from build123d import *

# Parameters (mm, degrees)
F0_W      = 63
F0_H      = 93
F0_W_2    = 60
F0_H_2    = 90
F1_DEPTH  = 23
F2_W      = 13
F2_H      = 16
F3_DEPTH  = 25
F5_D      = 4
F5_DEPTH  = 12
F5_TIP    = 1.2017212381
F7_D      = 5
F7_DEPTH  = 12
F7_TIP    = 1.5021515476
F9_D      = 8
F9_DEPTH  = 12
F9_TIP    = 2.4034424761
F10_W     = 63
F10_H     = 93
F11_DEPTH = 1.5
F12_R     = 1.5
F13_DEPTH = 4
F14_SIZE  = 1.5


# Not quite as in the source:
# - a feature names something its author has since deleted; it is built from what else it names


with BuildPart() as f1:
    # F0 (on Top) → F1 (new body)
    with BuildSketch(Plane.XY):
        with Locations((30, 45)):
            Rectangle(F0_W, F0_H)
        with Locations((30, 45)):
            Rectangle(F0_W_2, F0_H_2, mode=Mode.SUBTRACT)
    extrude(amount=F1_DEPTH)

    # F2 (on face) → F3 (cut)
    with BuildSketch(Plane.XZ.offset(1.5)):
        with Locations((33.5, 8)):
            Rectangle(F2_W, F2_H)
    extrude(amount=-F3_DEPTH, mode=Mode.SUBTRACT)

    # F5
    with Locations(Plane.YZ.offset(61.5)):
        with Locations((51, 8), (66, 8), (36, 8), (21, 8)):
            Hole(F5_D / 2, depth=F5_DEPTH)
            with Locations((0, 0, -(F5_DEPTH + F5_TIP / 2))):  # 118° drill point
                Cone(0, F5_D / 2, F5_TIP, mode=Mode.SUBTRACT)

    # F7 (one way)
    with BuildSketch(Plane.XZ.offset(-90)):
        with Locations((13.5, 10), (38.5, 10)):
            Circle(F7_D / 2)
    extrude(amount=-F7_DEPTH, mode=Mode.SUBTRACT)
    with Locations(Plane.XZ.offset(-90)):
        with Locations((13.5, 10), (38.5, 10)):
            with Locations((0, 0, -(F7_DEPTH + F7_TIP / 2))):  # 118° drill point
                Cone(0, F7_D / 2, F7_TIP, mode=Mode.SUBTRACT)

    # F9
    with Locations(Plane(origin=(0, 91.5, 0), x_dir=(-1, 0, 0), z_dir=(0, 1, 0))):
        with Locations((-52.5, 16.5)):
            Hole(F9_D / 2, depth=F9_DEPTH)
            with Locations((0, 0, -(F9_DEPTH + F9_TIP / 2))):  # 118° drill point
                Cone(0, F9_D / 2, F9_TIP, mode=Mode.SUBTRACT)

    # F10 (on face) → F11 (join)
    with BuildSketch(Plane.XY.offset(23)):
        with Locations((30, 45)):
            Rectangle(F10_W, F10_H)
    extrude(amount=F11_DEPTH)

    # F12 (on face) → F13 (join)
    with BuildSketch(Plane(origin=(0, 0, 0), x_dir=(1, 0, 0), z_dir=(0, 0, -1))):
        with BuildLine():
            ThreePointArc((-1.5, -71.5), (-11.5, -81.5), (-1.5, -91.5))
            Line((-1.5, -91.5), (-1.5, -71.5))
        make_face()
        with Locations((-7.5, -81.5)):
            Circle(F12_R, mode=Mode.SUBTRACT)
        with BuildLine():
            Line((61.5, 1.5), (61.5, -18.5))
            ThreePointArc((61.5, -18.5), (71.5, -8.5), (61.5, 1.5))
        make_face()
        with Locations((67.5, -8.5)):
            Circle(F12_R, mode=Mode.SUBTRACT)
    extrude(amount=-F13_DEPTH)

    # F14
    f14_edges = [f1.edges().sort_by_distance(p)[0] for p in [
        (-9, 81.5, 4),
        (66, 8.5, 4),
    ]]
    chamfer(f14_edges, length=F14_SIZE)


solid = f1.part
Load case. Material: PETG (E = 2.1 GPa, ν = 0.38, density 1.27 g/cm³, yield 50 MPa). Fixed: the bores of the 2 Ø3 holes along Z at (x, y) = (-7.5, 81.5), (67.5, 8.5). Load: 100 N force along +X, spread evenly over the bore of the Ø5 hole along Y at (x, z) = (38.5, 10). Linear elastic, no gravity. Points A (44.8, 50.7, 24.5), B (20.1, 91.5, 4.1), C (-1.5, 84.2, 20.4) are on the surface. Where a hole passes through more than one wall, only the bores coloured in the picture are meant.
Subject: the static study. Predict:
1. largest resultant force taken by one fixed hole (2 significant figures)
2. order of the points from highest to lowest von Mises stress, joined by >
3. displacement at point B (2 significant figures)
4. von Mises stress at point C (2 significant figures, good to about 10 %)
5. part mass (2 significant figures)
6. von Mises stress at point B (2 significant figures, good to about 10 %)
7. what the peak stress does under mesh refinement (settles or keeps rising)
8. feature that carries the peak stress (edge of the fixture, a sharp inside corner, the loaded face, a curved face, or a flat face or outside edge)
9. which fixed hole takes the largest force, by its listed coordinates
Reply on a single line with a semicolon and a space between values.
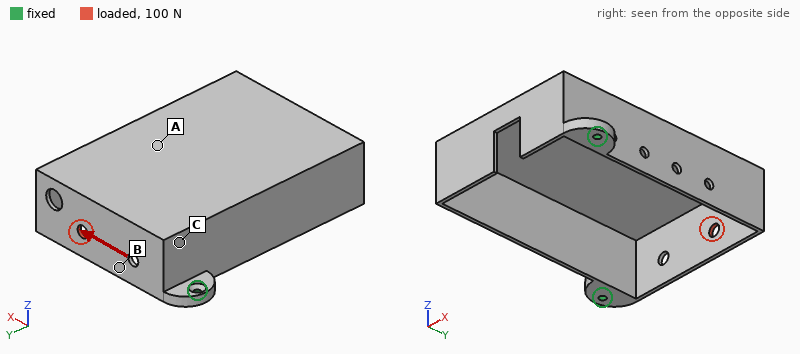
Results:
92 N; B > C > A; 0.63 mm; 2.0 MPa; 25 g; 5.2 MPa; keeps rising; edge of the fixture; (-7.5, 81.5)
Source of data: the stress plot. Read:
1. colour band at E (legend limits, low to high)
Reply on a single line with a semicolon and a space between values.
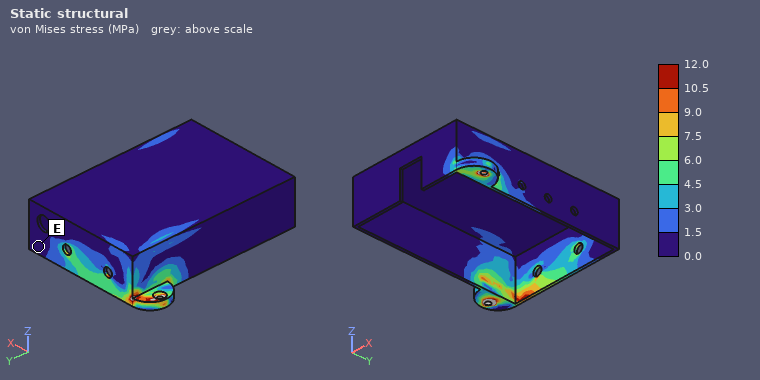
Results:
0.0 to 1.5 MPa
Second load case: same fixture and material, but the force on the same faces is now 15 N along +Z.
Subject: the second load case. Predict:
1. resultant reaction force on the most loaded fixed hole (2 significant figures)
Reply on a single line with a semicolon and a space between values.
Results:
13 N
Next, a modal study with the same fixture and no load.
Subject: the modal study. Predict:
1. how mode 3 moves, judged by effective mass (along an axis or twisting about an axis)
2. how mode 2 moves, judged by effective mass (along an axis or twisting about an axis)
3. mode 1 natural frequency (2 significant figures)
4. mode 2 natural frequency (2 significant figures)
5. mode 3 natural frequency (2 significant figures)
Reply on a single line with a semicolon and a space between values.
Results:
along X; along Z; 160 Hz; 440 Hz; 480 Hz
